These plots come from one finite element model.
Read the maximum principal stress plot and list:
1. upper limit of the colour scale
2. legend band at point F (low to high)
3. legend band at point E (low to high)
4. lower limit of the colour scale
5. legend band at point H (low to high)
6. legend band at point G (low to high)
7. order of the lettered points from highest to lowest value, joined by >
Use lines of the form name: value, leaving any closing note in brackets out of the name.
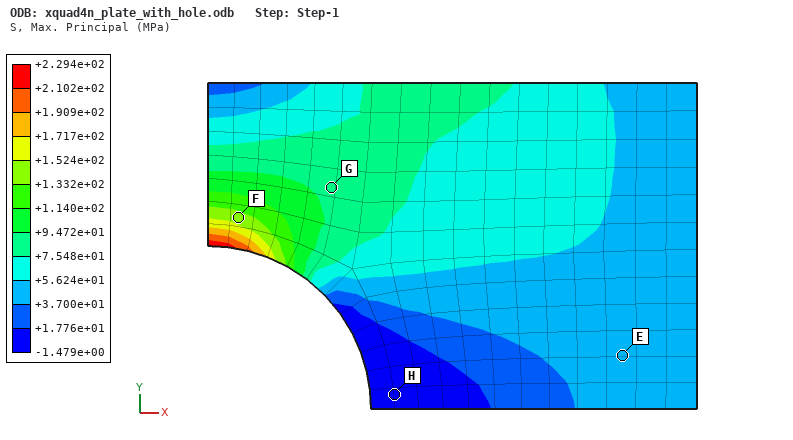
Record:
upper limit of the colour scale: +2.294e+02 MPa
legend band at point F: +1.332e+02 to +1.524e+02 MPa
legend band at point E: +3.700e+01 to +5.624e+01 MPa
lower limit of the colour scale: -1.479e+00 MPa
legend band at point H: -1.479e+00 to +1.776e+01 MPa
legend band at point G: +7.548e+01 to +9.472e+01 MPa
order of the lettered points from highest to lowest value, joined by >: F > G > E > H
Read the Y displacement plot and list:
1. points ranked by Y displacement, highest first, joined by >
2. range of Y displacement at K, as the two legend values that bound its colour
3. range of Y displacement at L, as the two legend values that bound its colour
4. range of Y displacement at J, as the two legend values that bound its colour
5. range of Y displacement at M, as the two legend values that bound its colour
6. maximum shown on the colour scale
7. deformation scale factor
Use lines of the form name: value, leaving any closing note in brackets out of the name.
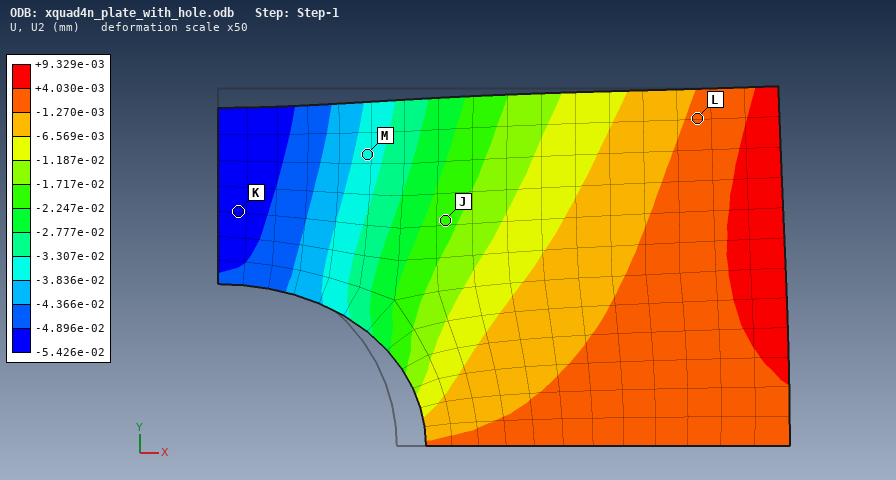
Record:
points ranked by Y displacement, highest first, joined by >: L > J > M > K
range of Y displacement at K, as the two legend values that bound its colour: -5.426e-02 to -4.896e-02 mm
range of Y displacement at L, as the two legend values that bound its colour: -1.270e-03 to +4.030e-03 mm
range of Y displacement at J, as the two legend values that bound its colour: -2.247e-02 to -1.717e-02 mm
range of Y displacement at M, as the two legend values that bound its colour: -3.836e-02 to -3.307e-02 mm
maximum shown on the colour scale: +9.329e-03 mm
deformation scale factor: 50
